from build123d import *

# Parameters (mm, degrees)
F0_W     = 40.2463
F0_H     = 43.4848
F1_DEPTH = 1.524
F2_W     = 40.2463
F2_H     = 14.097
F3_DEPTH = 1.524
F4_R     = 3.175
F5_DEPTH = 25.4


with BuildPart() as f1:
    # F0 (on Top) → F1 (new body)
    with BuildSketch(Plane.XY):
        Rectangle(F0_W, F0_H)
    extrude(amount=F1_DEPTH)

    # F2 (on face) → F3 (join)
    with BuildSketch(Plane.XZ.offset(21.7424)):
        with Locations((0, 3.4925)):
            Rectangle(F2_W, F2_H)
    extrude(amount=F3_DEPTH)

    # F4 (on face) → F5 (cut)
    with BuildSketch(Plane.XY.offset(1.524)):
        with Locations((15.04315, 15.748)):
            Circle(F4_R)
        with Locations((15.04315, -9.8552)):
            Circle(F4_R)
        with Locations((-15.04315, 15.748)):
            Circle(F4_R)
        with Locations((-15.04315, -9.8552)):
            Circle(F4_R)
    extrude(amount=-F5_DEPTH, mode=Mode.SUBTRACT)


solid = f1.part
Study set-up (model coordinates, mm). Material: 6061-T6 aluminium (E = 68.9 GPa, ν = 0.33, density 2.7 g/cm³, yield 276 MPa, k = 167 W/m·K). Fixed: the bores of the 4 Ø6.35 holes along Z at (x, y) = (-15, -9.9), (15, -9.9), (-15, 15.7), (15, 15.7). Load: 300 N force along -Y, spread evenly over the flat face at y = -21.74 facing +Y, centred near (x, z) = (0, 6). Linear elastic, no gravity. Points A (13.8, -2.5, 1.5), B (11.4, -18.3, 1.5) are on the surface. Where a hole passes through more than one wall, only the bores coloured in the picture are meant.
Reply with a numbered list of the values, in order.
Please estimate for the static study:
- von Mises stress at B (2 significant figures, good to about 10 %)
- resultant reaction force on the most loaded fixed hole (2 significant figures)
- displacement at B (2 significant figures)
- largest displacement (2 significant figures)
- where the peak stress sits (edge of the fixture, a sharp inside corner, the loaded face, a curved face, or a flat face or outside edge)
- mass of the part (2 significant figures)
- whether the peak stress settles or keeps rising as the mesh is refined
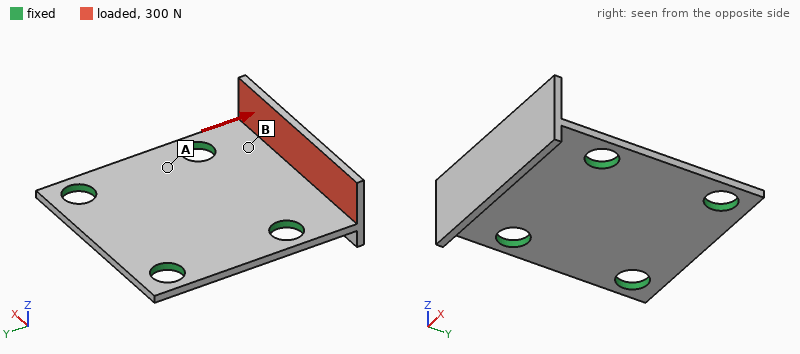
1. 97 MPa
2. 130 N
3. 0.043 mm
4. 0.26 mm
5. edge of the fixture
6. 9.0 g
7. keeps rising
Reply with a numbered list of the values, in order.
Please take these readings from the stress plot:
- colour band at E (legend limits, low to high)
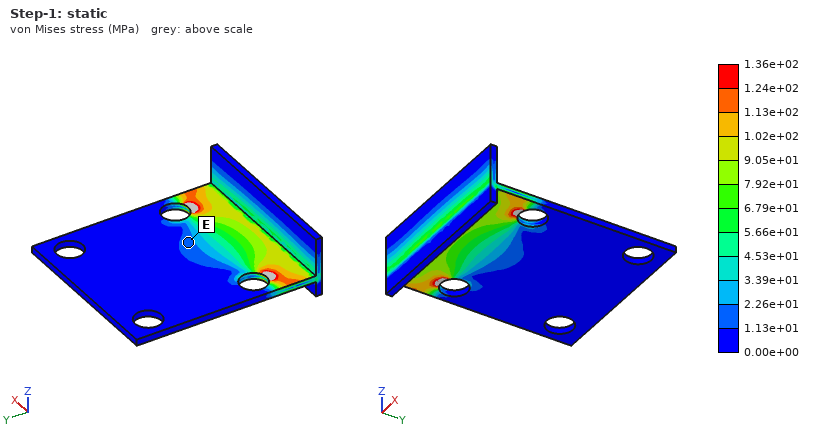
1. 1.13e+01 to 2.26e+01 MPa
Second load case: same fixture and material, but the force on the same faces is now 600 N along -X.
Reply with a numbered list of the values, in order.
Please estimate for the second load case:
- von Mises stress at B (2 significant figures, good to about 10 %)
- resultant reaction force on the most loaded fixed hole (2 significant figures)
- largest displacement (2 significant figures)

1. 71 MPa
2. 360 N
3. 0.15 mm
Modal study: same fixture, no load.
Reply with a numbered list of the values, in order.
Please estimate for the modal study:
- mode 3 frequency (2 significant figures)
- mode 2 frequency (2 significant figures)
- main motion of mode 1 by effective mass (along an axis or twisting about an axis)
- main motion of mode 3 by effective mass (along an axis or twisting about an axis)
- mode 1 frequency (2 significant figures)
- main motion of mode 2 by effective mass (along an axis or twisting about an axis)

1. 9900 Hz
2. 5800 Hz
3. along Z
4. along Z
5. 3600 Hz
6. twisting about Y
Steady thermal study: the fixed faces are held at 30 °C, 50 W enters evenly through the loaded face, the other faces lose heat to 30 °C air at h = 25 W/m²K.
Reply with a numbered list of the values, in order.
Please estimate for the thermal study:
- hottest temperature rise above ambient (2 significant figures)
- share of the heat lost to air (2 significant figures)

1. 83 K
2. 4.8 %
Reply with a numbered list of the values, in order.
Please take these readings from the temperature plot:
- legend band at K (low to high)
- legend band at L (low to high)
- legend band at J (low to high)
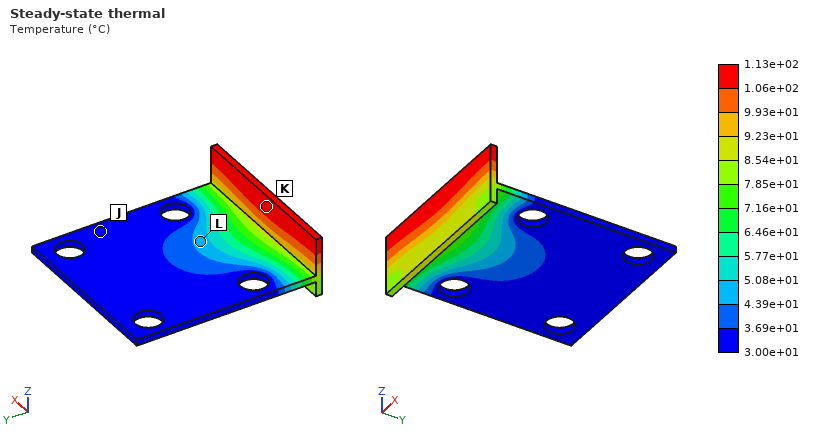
1. 1.06e+02 to 1.13e+02 °C
2. 4.39e+01 to 5.08e+01 °C
3. 3.00e+01 to 3.69e+01 °C
